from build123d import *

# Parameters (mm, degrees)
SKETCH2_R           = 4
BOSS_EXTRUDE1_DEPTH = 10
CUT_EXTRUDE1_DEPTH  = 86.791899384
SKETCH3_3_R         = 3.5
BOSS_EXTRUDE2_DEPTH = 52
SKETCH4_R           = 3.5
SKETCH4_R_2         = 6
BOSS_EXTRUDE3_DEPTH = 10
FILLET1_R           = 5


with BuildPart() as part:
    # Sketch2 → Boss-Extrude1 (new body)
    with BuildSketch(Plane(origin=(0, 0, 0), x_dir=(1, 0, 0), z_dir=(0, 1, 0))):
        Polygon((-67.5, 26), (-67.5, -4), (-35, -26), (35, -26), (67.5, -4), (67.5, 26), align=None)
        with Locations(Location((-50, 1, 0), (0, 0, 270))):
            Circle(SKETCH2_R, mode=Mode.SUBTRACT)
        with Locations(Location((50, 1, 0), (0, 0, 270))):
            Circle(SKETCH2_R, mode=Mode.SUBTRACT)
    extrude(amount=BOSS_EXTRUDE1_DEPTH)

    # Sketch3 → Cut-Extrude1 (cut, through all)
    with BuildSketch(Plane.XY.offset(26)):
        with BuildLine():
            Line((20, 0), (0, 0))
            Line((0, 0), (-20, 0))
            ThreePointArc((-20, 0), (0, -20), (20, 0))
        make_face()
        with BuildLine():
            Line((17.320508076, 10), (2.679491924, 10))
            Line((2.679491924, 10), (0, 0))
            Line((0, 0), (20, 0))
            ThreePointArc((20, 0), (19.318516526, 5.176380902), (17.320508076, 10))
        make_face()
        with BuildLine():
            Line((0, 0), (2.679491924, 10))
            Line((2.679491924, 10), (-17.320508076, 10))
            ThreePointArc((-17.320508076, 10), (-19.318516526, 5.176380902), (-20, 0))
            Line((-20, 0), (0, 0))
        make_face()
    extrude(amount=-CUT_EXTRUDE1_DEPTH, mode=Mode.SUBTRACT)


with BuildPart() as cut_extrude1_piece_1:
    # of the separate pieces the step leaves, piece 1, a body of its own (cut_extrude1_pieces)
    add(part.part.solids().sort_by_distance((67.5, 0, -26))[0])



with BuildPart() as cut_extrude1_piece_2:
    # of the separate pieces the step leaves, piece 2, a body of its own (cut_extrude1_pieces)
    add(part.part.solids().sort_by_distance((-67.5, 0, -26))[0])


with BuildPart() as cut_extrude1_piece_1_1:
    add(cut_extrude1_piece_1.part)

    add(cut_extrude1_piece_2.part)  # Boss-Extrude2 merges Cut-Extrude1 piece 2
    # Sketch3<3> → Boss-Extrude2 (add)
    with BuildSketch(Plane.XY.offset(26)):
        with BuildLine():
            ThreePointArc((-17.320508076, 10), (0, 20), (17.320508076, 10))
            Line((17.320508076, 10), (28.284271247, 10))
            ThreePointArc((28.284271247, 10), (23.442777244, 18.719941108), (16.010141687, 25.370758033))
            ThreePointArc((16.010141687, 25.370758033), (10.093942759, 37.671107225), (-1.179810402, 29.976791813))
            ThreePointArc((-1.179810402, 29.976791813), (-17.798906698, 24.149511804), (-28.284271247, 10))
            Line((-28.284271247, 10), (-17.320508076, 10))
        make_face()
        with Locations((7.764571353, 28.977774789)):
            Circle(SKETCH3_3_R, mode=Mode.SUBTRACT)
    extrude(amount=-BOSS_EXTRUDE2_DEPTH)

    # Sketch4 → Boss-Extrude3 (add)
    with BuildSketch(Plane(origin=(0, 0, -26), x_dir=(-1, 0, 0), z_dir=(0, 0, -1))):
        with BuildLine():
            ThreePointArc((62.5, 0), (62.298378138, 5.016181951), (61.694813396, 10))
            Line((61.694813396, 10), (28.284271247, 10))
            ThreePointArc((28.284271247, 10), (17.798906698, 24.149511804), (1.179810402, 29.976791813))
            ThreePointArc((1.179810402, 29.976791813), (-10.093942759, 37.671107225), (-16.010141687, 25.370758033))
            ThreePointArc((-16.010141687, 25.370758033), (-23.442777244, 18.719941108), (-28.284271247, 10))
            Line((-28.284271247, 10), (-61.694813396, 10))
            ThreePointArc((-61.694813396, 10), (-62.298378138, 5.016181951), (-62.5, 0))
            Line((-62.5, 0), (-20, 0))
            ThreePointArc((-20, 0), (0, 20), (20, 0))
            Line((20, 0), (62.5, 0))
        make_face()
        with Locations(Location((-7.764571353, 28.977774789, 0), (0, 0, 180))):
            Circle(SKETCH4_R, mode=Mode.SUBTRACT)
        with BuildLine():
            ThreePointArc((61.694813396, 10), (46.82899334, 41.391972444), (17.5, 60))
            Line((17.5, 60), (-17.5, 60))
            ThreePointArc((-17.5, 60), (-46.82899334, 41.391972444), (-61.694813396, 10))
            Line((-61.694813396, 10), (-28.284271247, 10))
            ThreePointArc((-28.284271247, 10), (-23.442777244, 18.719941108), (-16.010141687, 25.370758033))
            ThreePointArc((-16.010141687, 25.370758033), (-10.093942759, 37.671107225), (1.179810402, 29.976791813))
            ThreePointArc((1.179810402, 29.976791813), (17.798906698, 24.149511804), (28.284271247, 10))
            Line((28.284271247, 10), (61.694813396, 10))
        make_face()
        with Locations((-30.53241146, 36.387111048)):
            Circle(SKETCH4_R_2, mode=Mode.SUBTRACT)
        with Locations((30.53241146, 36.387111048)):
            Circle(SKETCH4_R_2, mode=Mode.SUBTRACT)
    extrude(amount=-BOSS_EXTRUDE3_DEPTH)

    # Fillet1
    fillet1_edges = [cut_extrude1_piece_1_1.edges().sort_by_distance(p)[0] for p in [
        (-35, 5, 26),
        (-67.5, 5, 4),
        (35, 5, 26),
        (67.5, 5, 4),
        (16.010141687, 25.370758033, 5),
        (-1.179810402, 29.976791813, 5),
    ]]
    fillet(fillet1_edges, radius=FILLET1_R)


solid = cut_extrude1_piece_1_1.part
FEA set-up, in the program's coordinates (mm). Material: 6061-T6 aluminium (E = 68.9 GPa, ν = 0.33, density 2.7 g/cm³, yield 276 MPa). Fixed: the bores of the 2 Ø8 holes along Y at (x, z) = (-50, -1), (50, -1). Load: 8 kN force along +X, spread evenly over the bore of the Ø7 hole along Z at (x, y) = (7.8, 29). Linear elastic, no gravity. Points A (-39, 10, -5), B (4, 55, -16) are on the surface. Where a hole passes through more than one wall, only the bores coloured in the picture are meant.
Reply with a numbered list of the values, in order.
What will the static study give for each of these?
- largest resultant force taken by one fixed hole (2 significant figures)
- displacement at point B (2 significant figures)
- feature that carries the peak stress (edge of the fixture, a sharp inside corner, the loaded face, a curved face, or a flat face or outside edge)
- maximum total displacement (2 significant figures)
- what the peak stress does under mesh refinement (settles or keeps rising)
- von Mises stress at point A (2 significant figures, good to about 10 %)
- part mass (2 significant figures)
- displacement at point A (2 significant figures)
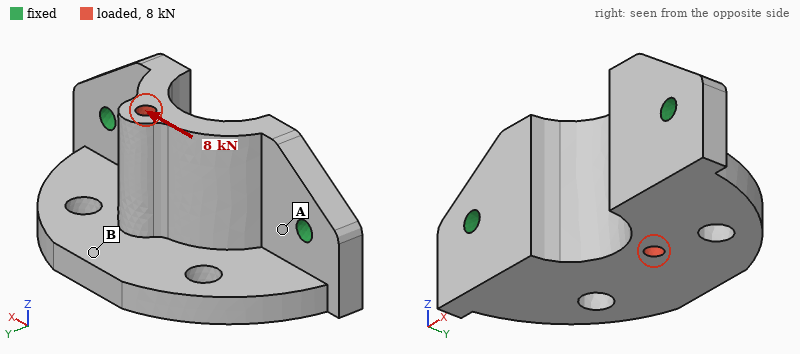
1. 4.6 kN
2. 17 µm
3. edge of the fixture
4. 26 µm
5. keeps rising
6. 21 MPa
7. 310 g
8. 4.4 µm
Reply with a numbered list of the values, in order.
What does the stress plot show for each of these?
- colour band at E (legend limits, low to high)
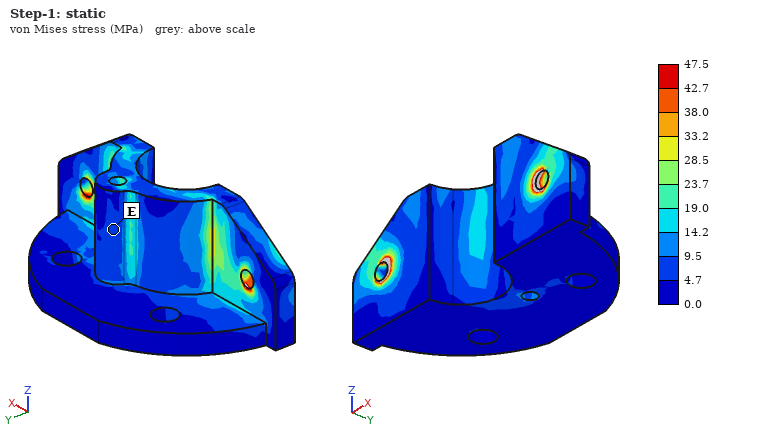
1. 4.7 to 9.5 MPa
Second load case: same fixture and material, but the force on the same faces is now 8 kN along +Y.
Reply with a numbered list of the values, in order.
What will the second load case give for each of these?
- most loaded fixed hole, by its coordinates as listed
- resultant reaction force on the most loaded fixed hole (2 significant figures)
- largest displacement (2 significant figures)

1. (50, -1)
2. 6.5 kN
3. 83 µm
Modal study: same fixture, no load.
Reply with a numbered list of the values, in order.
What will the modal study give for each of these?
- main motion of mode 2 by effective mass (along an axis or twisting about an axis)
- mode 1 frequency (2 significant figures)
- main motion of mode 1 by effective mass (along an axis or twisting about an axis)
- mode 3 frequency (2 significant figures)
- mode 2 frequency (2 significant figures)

1. along Y
2. 2100 Hz
3. along Z
4. 5700 Hz
5. 5400 Hz
